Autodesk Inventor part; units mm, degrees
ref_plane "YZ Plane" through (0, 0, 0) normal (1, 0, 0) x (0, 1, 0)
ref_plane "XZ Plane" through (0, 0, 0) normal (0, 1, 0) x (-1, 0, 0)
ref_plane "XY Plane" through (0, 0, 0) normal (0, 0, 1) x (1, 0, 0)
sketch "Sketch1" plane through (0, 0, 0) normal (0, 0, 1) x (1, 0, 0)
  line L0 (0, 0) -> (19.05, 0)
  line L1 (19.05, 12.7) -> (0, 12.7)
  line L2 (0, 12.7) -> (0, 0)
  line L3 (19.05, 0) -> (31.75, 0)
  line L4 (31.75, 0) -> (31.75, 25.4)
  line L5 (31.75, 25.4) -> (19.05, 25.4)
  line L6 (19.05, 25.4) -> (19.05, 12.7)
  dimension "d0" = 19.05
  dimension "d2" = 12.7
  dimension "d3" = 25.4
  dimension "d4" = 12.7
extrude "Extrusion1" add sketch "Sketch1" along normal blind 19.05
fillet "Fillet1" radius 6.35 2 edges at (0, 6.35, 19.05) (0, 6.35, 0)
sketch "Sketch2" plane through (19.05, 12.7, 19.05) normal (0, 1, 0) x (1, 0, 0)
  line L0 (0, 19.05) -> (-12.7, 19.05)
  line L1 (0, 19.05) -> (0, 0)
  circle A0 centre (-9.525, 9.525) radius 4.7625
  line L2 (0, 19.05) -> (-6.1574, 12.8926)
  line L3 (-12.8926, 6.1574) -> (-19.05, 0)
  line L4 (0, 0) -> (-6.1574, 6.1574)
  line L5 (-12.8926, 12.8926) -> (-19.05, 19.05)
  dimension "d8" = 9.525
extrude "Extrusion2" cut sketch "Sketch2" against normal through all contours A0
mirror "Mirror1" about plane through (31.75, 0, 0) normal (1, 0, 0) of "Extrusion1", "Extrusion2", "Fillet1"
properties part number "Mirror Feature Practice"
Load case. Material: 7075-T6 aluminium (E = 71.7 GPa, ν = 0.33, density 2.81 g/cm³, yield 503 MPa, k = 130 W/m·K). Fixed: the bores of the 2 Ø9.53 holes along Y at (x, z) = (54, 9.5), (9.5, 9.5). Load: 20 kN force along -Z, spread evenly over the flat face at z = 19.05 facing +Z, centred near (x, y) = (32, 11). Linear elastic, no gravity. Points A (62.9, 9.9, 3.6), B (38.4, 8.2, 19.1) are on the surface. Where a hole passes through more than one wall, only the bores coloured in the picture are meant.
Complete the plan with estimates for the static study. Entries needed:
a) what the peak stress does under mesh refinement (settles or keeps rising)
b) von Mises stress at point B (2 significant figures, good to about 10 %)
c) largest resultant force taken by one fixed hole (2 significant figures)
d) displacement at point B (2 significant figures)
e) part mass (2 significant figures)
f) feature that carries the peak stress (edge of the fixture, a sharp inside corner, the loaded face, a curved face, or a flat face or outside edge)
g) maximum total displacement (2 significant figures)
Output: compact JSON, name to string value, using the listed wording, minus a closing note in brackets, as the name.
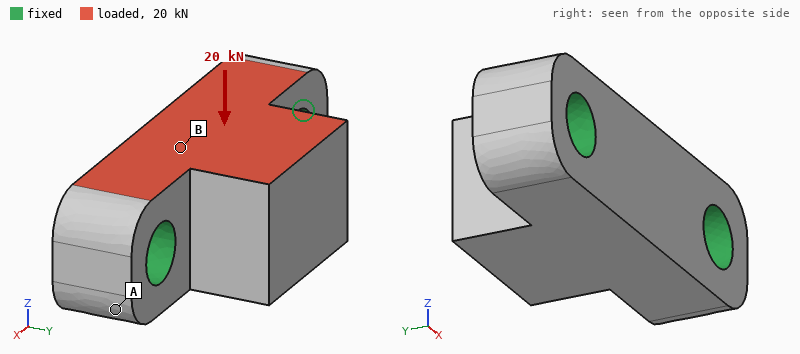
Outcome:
{"what the peak stress does under mesh refinement": "keeps rising", "von Mises stress at point B": "63 MPa", "largest resultant force taken by one fixed hole": "10 kN", "displacement at point B": "30 µm", "part mass": "54 g", "feature that carries the peak stress": "edge of the fixture", "maximum total displacement": "70 µm"}
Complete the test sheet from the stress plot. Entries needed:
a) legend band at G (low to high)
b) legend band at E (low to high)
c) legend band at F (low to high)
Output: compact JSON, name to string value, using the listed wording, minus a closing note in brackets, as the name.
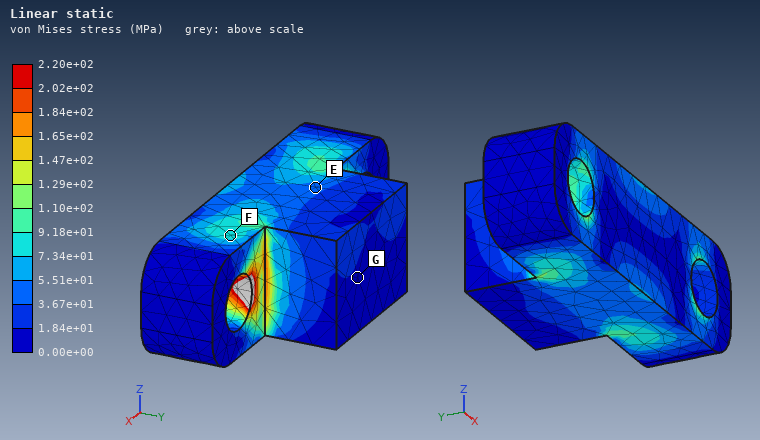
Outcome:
{"legend band at G": "0.00e+00 to 1.84e+01 MPa", "legend band at E": "3.67e+01 to 5.51e+01 MPa", "legend band at F": "7.34e+01 to 9.18e+01 MPa"}
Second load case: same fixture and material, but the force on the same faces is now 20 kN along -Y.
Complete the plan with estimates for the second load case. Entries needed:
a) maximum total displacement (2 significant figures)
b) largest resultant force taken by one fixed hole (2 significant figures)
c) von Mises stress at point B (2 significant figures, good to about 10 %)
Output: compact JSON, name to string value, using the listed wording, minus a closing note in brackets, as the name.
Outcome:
{"maximum total displacement": "91 µm", "largest resultant force taken by one fixed hole": "10 kN", "von Mises stress at point B": "63 MPa"}
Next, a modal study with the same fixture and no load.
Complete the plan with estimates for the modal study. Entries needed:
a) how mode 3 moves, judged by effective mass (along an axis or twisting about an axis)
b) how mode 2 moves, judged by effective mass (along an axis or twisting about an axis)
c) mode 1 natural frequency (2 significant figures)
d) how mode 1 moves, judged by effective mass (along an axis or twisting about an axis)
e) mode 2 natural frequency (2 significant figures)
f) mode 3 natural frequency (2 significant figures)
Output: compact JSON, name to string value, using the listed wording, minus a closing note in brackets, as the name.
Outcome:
{"how mode 3 moves, judged by effective mass": "along X", "how mode 2 moves, judged by effective mass": "along Y", "mode 1 natural frequency": "14 kHz", "how mode 1 moves, judged by effective mass": "along Z", "mode 2 natural frequency": "24 kHz", "mode 3 natural frequency": "29 kHz"}
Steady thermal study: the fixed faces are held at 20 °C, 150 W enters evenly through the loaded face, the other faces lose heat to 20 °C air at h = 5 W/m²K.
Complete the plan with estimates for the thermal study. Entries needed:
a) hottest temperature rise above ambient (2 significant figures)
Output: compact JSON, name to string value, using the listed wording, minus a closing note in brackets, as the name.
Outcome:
{"hottest temperature rise above ambient": "34 K"}
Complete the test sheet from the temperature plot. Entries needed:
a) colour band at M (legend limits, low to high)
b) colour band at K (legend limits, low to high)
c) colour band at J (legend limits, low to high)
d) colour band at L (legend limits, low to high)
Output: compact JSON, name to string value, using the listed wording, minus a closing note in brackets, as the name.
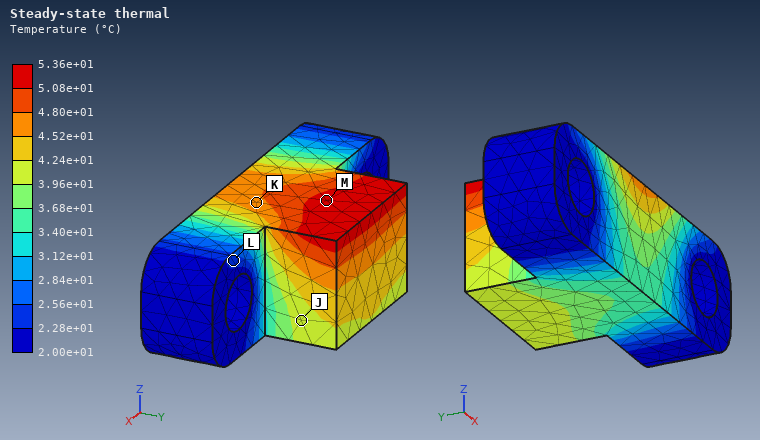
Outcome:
{"colour band at M": "5.08e+01 to 5.36e+01 °C", "colour band at K": "4.52e+01 to 4.80e+01 °C", "colour band at J": "3.96e+01 to 4.24e+01 °C", "colour band at L": "2.28e+01 to 2.56e+01 °C"}
